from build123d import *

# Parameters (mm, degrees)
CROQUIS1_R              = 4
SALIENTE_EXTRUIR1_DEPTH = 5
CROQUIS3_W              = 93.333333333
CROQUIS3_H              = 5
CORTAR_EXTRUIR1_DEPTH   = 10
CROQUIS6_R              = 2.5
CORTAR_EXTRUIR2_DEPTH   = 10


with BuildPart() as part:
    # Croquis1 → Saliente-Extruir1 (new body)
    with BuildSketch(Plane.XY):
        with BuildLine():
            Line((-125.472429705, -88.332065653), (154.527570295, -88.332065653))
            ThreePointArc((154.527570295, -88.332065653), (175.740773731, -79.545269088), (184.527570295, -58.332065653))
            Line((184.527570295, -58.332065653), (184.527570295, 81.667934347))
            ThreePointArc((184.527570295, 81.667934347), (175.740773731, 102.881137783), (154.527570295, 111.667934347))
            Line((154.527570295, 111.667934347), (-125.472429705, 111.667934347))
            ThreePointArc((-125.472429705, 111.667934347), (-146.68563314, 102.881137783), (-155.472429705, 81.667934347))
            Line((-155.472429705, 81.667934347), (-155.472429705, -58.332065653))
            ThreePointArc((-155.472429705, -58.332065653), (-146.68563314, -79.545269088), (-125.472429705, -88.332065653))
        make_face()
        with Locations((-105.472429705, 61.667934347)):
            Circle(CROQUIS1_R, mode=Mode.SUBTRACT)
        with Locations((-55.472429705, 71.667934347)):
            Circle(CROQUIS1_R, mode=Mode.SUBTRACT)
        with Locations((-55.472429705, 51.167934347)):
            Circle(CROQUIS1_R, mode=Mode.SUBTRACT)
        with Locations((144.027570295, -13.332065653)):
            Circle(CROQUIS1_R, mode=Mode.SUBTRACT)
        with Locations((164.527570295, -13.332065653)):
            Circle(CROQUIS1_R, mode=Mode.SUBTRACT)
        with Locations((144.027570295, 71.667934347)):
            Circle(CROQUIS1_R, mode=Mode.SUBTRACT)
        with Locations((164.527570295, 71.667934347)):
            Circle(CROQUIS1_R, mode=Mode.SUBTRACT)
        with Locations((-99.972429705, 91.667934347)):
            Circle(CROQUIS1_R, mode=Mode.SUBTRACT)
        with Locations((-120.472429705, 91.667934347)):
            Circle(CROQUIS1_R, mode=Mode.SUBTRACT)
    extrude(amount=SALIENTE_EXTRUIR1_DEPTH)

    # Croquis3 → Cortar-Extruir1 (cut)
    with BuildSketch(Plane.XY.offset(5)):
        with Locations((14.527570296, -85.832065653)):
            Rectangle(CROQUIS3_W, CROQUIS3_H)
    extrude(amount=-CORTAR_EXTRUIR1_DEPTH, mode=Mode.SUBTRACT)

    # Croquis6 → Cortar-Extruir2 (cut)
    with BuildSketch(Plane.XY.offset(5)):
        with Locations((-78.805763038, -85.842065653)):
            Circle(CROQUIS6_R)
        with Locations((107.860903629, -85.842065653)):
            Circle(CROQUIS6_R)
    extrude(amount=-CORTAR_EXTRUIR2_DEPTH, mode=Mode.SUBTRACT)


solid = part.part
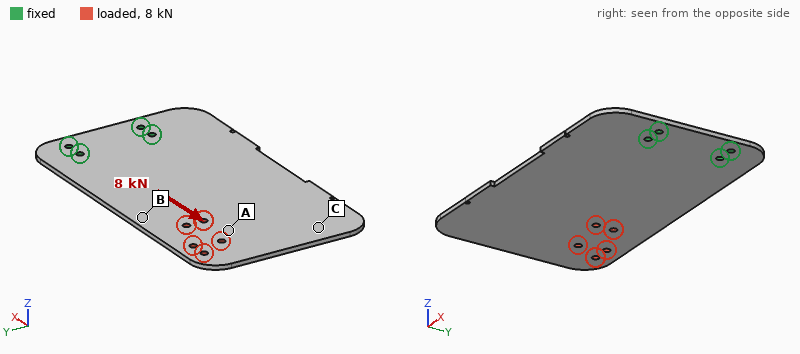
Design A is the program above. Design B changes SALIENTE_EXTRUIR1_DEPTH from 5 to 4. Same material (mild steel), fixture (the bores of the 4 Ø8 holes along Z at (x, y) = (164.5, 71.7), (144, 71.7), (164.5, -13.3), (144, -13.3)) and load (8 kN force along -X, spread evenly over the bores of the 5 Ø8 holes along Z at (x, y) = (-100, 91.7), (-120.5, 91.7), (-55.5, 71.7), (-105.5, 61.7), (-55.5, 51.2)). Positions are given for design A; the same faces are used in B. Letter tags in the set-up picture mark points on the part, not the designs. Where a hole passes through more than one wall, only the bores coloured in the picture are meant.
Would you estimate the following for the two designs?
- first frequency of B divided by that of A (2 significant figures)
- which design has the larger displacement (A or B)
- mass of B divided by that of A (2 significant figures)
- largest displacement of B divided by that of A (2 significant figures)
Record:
0.80
B
0.80
1.3
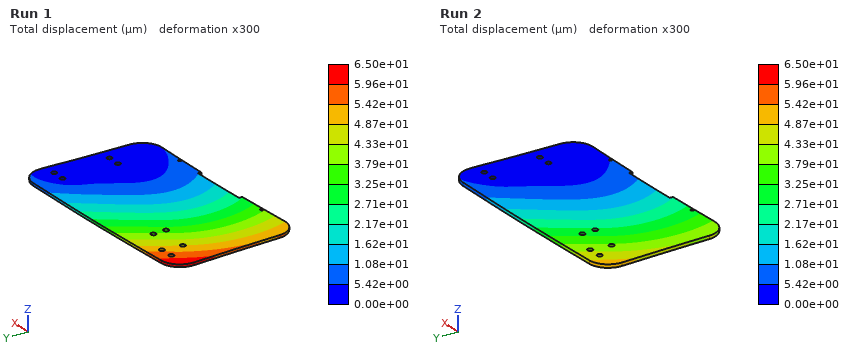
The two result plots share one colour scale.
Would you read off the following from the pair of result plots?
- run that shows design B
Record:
Run 1
